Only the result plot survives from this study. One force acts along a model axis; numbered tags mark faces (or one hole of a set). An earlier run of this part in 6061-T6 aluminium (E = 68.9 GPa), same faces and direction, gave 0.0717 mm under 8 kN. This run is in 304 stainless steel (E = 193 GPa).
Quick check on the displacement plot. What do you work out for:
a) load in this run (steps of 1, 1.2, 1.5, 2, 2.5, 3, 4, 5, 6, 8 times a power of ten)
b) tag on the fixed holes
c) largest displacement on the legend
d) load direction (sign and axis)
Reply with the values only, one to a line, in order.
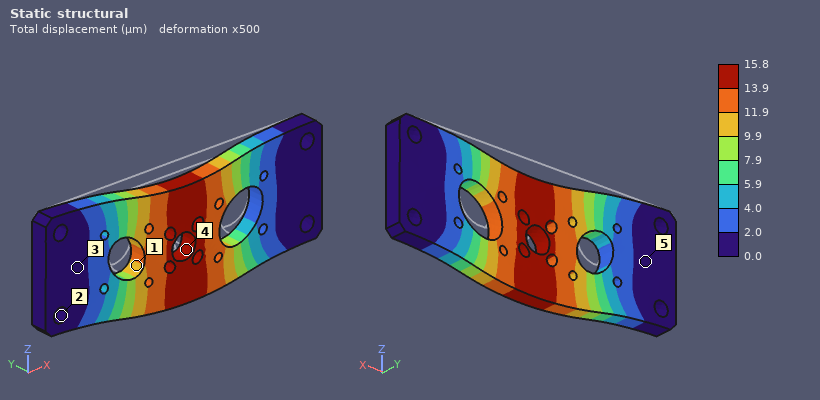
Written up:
5 kN
2
15.8 µm
-Z
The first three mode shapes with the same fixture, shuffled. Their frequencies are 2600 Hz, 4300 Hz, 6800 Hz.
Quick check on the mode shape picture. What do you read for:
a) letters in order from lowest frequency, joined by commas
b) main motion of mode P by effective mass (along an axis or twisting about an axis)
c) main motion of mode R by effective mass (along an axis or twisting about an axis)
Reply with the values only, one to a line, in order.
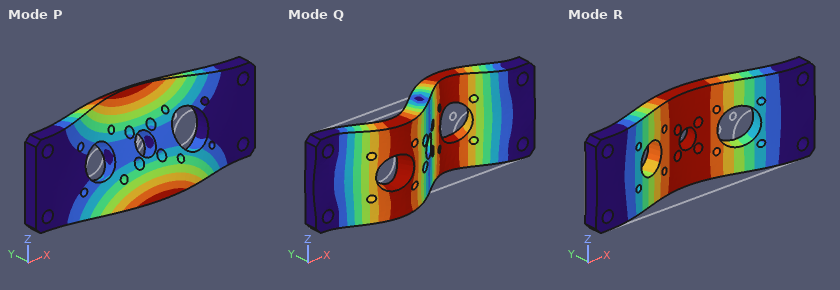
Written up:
R, P, Q
twisting about X
along Y
